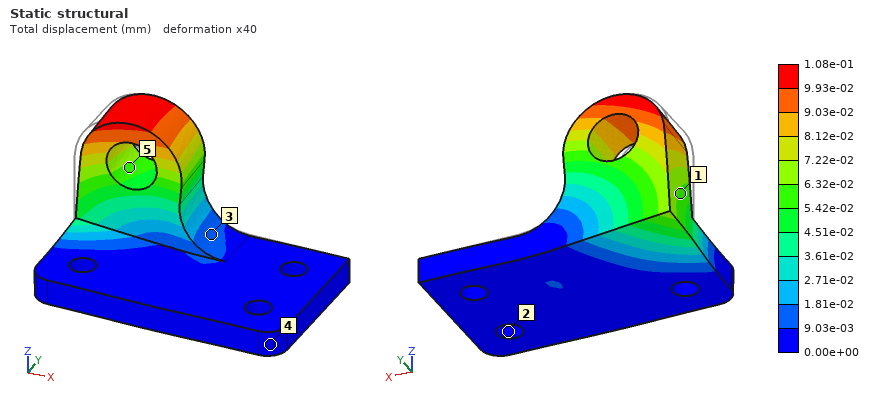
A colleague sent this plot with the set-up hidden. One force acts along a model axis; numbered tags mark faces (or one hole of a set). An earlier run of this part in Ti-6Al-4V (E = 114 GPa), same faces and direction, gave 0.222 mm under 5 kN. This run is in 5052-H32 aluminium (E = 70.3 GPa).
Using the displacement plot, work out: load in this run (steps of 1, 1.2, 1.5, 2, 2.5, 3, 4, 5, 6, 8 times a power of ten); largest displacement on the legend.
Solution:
1.5 kN
1.08e-01 mm
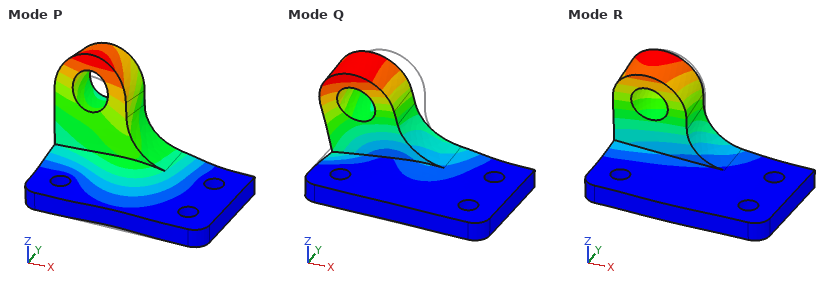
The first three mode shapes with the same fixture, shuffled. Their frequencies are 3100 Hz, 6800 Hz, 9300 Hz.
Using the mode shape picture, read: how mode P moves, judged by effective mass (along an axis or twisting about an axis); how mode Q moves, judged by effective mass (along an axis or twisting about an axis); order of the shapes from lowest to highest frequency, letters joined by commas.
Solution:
along Z
along X
R, Q, P
